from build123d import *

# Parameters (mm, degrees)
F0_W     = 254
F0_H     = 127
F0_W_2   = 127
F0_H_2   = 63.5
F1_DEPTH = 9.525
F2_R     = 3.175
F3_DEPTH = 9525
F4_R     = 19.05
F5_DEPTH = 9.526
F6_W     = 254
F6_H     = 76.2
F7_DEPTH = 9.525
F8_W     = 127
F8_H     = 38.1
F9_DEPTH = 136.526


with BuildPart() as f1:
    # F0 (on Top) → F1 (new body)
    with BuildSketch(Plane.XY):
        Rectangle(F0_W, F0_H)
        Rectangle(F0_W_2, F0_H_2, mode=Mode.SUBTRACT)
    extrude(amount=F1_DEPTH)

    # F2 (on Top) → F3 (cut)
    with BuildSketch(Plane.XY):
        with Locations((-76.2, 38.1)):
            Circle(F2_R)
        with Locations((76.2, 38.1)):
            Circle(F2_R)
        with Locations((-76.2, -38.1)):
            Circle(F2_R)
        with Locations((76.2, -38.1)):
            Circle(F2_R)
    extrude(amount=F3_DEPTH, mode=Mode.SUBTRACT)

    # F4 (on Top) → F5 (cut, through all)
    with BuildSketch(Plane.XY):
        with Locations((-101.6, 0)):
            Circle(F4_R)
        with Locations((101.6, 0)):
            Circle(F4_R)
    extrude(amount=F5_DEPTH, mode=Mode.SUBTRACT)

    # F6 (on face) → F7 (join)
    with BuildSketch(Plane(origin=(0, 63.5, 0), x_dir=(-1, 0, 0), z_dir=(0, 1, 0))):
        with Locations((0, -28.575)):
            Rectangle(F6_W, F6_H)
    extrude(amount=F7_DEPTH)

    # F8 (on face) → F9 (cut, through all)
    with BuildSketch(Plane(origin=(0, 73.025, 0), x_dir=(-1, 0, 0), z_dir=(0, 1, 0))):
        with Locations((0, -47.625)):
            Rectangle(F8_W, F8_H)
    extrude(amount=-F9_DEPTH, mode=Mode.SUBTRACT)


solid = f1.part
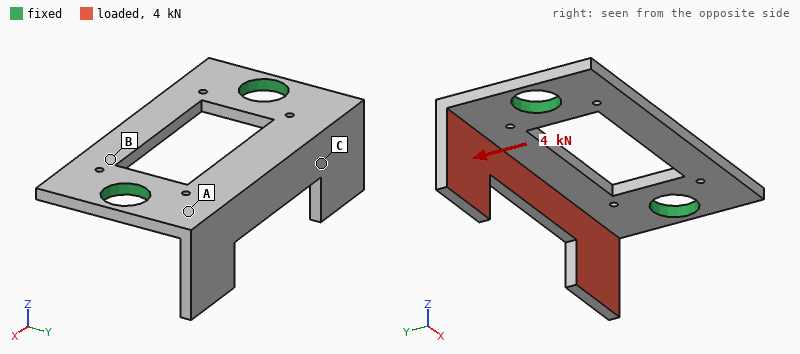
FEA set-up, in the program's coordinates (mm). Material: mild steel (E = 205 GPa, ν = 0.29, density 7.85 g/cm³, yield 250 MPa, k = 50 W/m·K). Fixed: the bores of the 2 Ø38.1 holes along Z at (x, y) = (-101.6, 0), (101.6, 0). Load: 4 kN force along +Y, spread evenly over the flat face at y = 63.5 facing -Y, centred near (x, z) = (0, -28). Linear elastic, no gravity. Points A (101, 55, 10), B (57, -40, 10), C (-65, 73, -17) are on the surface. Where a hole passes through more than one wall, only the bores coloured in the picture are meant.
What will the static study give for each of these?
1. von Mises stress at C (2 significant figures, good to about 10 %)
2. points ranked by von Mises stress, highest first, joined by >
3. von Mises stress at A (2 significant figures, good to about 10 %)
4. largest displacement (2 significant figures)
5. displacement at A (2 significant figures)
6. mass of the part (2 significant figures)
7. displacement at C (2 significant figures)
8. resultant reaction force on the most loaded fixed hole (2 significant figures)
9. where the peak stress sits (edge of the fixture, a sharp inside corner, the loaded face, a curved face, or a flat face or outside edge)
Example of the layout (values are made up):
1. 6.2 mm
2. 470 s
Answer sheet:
1. 20 MPa
2. A > C > B
3. 45 MPa
4. 0.29 mm
5. 0.052 mm
6. 2.7 kg
7. 0.13 mm
8. 2.0 kN
9. a curved face
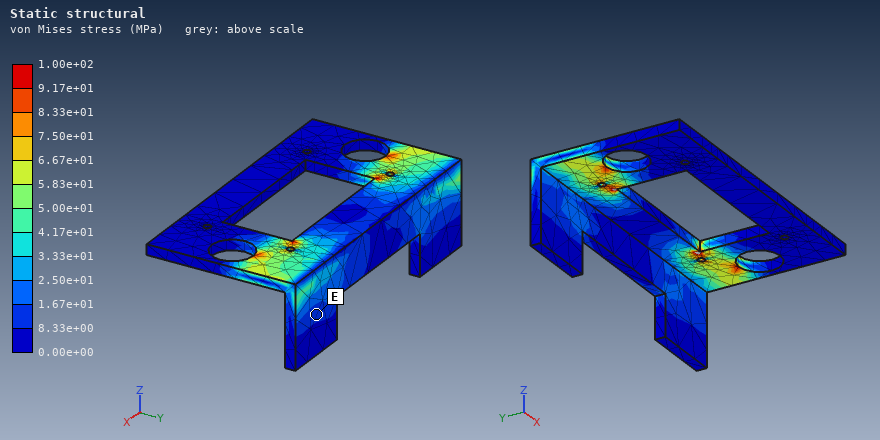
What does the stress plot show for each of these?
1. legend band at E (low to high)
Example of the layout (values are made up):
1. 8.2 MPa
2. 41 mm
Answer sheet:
1. 8.33e+00 to 1.67e+01 MPa
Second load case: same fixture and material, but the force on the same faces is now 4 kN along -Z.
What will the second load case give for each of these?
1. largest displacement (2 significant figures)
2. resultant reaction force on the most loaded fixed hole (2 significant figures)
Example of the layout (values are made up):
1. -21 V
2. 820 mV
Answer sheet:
1. 0.19 mm
2. 2.0 kN
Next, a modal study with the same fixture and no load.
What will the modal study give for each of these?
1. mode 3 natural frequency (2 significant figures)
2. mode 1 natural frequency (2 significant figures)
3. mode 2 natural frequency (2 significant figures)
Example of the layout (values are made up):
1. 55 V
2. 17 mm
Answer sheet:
1. 1300 Hz
2. 640 Hz
3. 910 Hz
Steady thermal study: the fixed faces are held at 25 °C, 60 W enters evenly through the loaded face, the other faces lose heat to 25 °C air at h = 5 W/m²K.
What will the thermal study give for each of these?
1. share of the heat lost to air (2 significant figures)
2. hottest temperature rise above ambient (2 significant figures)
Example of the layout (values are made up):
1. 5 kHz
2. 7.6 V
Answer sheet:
1. 15 %
2. 62 K
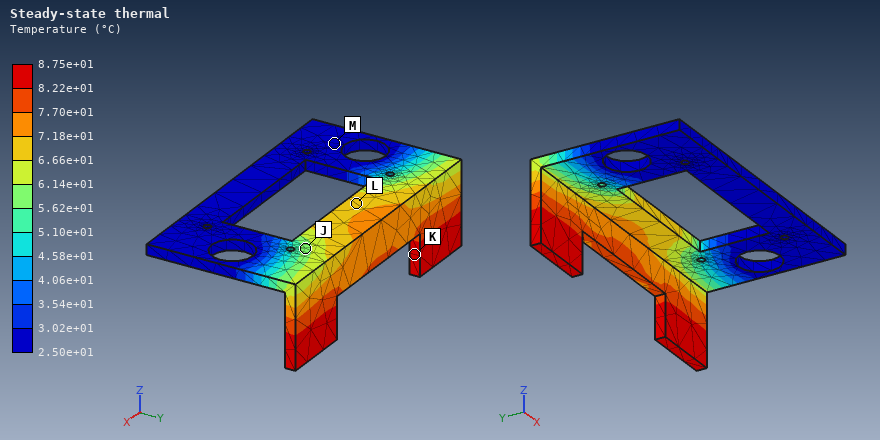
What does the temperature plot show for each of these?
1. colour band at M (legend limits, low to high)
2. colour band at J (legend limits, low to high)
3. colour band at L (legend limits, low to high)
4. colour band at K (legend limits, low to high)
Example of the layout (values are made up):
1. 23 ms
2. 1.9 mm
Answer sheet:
1. 2.50e+01 to 3.02e+01 °C
2. 5.62e+01 to 6.14e+01 °C
3. 6.66e+01 to 7.18e+01 °C
4. 8.22e+01 to 8.75e+01 °C
